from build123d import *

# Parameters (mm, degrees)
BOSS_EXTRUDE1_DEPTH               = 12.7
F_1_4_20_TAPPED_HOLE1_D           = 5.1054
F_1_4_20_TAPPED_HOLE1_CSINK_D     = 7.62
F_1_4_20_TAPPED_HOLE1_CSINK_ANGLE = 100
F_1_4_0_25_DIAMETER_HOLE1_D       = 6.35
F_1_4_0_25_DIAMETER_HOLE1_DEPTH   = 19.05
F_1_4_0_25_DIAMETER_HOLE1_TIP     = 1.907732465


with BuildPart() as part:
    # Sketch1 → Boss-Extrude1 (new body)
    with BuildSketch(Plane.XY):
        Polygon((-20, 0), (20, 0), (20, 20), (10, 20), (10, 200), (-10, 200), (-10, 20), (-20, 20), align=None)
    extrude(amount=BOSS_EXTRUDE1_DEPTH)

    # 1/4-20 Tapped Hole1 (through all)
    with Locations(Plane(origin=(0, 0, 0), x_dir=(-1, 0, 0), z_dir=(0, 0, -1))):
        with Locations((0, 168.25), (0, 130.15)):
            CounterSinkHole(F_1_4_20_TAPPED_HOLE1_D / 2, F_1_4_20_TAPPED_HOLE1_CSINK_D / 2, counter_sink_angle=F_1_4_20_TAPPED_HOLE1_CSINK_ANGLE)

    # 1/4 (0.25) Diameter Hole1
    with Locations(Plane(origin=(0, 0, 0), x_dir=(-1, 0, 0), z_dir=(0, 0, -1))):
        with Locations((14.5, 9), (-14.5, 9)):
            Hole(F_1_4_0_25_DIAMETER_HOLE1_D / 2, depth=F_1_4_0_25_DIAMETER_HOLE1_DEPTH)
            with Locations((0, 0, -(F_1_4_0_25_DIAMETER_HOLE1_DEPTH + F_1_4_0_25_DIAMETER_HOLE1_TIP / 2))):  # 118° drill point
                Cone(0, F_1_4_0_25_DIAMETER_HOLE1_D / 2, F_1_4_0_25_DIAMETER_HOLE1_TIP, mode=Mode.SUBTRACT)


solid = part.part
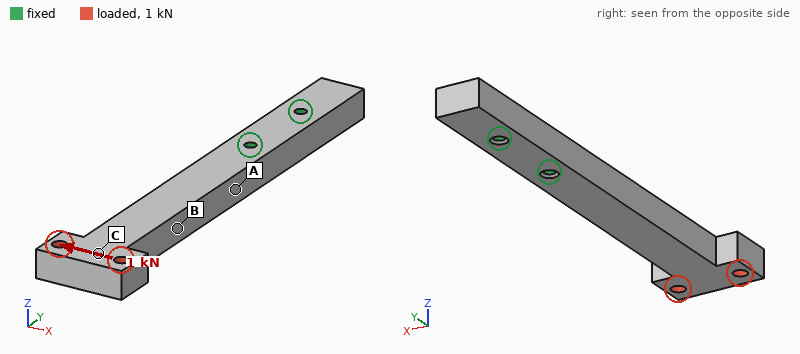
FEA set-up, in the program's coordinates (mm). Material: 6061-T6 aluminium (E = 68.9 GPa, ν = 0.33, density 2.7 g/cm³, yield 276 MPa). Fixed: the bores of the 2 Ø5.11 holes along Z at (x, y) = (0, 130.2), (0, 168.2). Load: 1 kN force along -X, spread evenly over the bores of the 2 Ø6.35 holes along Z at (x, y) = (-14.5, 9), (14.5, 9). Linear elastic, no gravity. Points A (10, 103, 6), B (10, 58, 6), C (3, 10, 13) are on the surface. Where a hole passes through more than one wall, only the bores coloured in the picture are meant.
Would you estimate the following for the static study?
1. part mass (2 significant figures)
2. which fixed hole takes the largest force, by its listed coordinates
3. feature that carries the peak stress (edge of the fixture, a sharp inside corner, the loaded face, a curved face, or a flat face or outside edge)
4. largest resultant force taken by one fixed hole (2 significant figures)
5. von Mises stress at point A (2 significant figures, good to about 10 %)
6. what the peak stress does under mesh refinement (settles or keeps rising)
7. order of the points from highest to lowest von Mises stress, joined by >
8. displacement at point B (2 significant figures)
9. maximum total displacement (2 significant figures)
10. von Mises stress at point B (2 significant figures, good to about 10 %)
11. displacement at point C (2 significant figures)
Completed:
150 g
(0, 130.2)
edge of the fixture
3.0 kN
110 MPa
keeps rising
A > B > C
0.58 mm
1.4 mm
58 MPa
1.2 mm
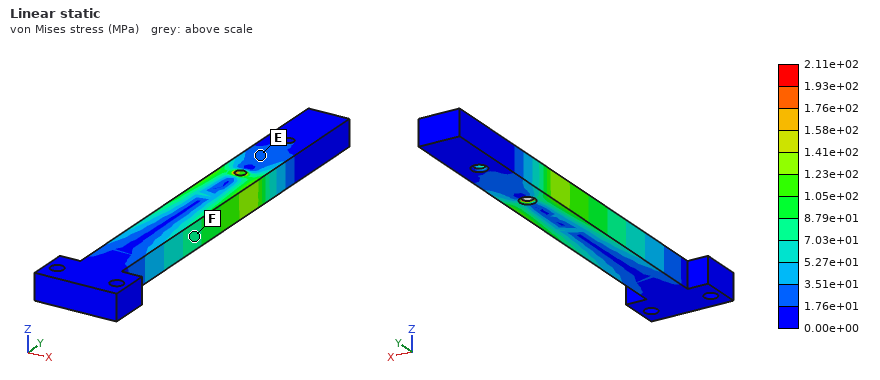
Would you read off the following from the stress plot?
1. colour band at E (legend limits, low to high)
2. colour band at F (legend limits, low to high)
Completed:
1.76e+01 to 3.51e+01 MPa
7.03e+01 to 8.79e+01 MPa
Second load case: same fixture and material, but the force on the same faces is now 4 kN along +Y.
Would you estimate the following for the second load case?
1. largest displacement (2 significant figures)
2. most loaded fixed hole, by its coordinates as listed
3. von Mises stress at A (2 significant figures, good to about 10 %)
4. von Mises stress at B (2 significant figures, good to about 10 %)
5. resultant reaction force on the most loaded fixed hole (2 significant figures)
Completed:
34 µm
(0, 130.2)
16 MPa
16 MPa
3.7 kN
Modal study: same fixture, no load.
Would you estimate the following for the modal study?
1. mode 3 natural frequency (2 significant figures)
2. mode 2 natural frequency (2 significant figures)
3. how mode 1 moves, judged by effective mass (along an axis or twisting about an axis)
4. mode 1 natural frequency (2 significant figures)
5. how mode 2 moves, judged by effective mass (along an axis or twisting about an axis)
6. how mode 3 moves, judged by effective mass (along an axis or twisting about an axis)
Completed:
3200 Hz
710 Hz
along Z
500 Hz
along X
twisting about Y
